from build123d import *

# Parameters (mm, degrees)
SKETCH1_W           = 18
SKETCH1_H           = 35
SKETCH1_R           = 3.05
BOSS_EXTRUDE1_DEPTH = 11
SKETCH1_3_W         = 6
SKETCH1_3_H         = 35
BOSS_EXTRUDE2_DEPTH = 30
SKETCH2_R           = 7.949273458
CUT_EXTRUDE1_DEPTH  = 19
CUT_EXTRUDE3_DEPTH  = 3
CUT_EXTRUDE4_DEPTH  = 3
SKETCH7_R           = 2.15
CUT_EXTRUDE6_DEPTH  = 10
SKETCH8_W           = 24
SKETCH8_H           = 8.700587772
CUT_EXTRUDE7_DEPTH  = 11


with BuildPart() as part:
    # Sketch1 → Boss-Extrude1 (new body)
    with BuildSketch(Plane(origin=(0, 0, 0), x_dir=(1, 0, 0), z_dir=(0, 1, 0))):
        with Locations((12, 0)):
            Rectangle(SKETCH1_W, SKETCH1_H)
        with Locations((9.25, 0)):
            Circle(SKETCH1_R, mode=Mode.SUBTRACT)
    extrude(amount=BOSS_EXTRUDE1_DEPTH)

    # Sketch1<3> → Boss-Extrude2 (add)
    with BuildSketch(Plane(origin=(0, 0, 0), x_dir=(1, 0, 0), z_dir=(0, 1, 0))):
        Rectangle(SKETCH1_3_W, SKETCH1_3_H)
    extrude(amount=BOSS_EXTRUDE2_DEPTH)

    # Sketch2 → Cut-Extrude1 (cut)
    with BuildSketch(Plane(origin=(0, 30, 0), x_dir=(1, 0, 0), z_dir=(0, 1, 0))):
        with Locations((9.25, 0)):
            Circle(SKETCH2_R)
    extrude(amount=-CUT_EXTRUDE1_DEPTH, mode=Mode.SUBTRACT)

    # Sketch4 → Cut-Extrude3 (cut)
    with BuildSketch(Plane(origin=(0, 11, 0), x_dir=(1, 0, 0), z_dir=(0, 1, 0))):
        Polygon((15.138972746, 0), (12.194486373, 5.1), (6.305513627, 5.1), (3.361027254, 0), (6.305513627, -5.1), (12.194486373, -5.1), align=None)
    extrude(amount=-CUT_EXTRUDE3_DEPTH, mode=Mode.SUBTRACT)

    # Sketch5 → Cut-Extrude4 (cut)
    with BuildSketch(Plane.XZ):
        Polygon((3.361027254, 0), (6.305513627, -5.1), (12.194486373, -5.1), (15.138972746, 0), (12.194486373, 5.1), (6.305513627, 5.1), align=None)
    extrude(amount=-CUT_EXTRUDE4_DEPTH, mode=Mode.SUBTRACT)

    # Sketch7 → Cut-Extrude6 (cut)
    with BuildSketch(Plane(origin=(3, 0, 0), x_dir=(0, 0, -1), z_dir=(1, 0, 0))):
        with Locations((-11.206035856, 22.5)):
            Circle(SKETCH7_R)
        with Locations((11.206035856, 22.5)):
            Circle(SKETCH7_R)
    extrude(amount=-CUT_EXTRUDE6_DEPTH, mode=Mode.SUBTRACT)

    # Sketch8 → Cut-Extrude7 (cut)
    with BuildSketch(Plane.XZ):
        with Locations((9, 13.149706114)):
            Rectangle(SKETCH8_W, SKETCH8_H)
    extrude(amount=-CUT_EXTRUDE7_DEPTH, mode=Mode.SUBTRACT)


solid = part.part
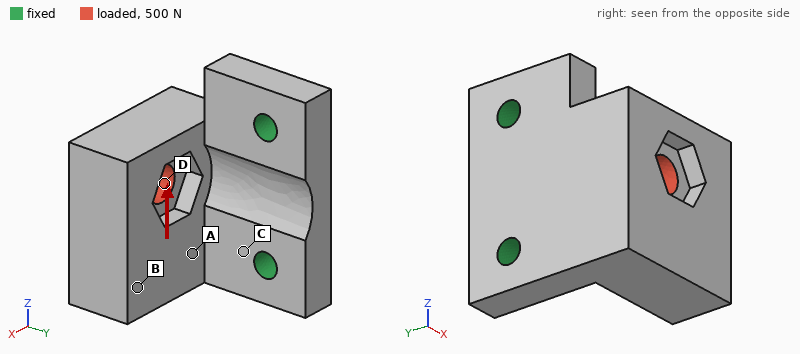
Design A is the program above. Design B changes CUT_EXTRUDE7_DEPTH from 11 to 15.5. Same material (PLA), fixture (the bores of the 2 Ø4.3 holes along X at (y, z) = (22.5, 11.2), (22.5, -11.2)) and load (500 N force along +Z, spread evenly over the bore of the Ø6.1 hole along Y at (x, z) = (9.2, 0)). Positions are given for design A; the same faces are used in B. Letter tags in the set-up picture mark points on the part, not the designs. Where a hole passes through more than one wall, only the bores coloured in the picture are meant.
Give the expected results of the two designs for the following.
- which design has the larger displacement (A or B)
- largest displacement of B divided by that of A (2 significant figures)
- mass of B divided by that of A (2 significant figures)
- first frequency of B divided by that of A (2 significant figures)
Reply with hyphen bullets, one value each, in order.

- B
- 1.2
- 0.98
- 0.95
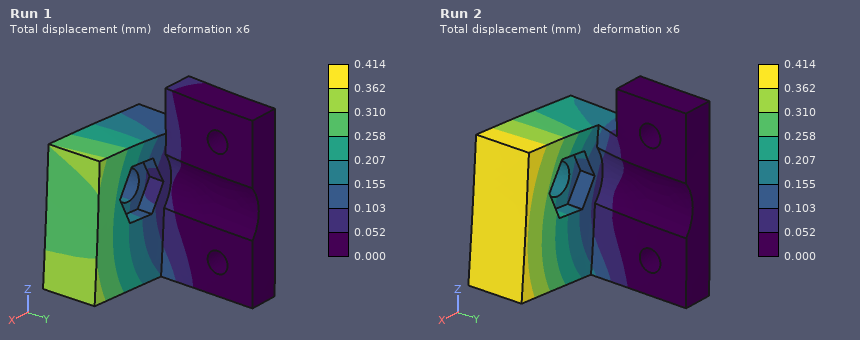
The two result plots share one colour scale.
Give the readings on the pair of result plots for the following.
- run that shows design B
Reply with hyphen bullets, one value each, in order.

- Run 2
